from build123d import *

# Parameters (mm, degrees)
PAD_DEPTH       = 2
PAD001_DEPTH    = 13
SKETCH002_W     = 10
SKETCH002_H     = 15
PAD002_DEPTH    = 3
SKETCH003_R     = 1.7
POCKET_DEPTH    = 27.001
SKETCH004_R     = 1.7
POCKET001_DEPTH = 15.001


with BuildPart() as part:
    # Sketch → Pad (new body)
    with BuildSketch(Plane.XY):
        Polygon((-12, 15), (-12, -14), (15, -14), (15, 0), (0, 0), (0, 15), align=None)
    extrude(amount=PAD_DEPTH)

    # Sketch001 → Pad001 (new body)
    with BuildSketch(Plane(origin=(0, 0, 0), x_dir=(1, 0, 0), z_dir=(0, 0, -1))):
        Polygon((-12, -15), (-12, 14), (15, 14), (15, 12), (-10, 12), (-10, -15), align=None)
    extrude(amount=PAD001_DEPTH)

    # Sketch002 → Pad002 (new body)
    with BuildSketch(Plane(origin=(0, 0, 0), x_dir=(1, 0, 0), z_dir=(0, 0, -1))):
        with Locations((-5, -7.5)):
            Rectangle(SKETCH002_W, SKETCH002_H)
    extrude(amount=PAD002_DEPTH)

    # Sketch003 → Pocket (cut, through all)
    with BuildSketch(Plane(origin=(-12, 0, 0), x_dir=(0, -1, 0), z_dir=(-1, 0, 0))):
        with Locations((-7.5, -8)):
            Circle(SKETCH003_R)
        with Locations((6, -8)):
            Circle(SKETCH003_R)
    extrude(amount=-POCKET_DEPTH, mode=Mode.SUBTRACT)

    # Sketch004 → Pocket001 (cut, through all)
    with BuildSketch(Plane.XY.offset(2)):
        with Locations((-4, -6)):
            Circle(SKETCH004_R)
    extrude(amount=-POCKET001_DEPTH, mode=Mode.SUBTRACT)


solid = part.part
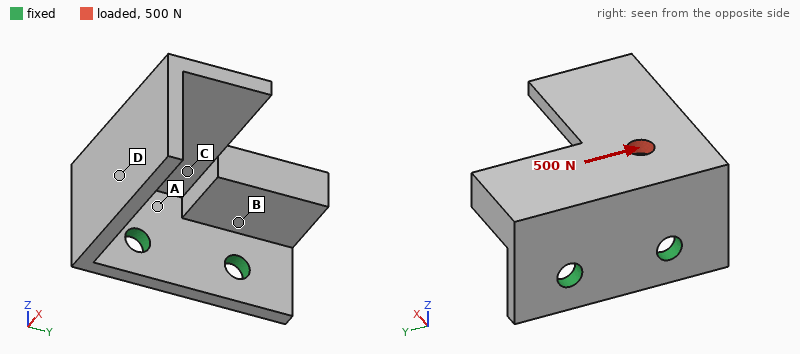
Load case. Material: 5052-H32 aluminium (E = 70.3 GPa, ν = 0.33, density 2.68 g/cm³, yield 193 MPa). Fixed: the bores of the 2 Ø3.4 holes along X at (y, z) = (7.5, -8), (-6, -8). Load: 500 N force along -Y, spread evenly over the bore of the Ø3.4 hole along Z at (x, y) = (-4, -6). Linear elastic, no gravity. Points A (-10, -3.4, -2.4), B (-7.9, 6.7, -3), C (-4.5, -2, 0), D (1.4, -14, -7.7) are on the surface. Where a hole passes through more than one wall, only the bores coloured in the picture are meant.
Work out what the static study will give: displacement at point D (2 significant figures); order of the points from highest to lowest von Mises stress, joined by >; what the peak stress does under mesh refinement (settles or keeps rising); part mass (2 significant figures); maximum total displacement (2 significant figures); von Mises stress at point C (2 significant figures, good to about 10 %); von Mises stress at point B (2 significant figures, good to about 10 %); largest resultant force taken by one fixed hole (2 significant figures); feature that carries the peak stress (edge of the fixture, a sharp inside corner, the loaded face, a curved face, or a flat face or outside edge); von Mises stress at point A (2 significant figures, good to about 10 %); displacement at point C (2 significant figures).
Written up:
42 µm
A > C > B > D
keeps rising
7.8 g
84 µm
39 MPa
21 MPa
420 N
edge of the fixture
51 MPa
20 µm
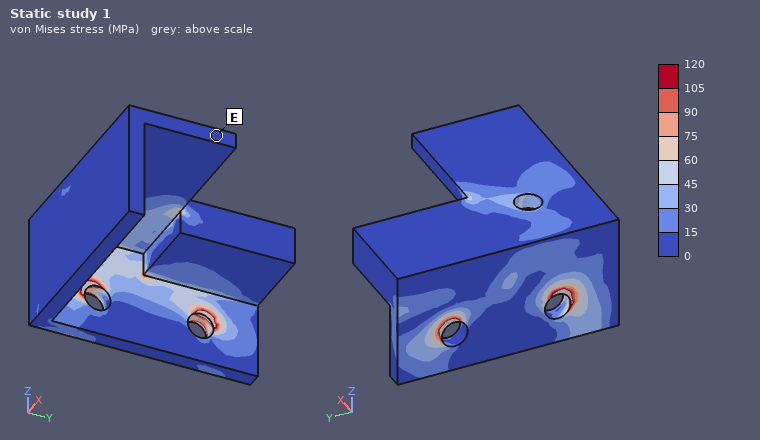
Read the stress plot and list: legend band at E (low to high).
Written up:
0 to 15 MPa
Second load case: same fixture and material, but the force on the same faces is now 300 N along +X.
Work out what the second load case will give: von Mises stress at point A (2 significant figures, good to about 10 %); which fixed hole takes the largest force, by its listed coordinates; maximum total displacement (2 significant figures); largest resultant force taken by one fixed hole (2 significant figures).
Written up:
39 MPa
(-6, -8)
0.16 mm
260 N
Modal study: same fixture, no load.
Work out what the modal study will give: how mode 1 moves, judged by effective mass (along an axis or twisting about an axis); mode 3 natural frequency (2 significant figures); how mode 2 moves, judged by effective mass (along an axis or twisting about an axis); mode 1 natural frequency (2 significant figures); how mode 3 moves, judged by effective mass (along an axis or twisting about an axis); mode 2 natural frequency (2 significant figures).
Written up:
along Z
9200 Hz
along Y
2900 Hz
along X
4300 Hz
